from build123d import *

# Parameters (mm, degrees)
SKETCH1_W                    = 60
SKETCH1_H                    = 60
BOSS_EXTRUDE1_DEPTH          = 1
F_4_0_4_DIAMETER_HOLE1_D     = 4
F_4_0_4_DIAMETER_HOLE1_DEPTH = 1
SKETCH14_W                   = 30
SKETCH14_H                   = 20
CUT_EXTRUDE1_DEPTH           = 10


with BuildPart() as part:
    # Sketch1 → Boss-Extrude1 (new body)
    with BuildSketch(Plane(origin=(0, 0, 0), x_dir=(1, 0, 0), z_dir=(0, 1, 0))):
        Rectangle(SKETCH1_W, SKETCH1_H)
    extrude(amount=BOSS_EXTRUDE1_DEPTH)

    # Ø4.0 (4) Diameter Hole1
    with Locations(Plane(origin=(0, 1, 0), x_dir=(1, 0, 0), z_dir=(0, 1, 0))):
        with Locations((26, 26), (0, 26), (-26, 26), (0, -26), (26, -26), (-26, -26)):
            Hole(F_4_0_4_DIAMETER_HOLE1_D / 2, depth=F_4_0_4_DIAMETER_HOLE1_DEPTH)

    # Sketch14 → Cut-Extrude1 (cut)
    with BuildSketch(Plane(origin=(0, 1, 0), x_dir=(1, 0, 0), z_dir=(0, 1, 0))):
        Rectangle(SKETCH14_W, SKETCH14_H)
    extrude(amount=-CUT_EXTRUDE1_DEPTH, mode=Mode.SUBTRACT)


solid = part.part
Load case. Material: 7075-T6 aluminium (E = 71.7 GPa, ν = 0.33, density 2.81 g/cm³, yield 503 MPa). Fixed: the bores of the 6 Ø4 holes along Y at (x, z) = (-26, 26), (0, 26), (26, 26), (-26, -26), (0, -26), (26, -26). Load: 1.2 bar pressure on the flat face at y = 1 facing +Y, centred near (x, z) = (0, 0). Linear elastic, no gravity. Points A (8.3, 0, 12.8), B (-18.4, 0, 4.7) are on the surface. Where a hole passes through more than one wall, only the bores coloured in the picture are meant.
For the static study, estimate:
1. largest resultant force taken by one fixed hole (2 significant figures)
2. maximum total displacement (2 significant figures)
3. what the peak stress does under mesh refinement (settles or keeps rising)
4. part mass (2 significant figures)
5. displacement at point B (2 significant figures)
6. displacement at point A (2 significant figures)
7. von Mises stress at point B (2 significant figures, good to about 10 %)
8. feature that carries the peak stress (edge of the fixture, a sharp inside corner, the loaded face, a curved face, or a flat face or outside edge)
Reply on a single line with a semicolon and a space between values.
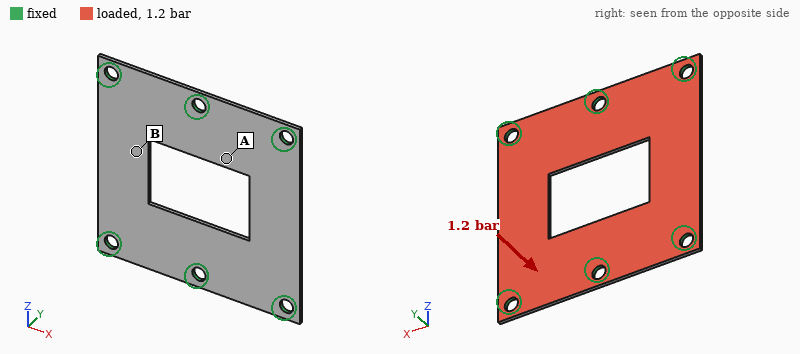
70 N; 0.33 mm; keeps rising; 8.2 g; 0.30 mm; 0.18 mm; 60 MPa; edge of the fixture
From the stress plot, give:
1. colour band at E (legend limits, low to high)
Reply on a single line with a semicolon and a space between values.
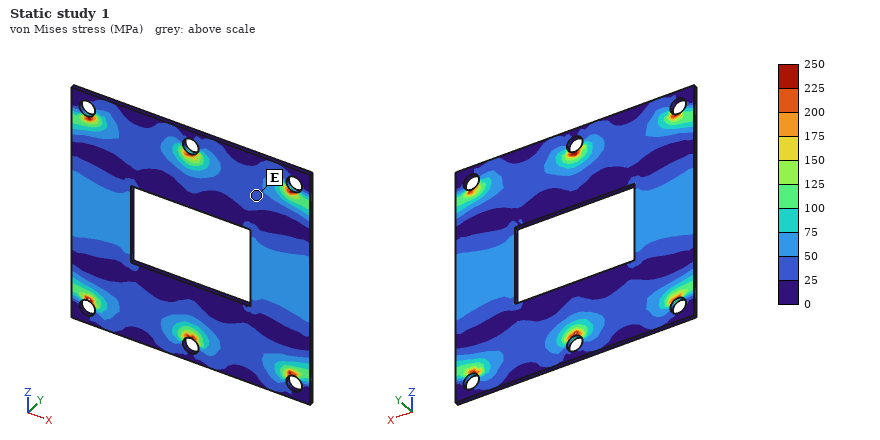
25 to 50 MPa
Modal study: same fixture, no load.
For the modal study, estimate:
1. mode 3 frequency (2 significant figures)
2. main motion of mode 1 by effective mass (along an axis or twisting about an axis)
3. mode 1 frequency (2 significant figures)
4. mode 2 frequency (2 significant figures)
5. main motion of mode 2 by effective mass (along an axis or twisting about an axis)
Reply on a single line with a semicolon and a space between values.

4200 Hz; along Y; 2200 Hz; 2300 Hz; twisting about Z
